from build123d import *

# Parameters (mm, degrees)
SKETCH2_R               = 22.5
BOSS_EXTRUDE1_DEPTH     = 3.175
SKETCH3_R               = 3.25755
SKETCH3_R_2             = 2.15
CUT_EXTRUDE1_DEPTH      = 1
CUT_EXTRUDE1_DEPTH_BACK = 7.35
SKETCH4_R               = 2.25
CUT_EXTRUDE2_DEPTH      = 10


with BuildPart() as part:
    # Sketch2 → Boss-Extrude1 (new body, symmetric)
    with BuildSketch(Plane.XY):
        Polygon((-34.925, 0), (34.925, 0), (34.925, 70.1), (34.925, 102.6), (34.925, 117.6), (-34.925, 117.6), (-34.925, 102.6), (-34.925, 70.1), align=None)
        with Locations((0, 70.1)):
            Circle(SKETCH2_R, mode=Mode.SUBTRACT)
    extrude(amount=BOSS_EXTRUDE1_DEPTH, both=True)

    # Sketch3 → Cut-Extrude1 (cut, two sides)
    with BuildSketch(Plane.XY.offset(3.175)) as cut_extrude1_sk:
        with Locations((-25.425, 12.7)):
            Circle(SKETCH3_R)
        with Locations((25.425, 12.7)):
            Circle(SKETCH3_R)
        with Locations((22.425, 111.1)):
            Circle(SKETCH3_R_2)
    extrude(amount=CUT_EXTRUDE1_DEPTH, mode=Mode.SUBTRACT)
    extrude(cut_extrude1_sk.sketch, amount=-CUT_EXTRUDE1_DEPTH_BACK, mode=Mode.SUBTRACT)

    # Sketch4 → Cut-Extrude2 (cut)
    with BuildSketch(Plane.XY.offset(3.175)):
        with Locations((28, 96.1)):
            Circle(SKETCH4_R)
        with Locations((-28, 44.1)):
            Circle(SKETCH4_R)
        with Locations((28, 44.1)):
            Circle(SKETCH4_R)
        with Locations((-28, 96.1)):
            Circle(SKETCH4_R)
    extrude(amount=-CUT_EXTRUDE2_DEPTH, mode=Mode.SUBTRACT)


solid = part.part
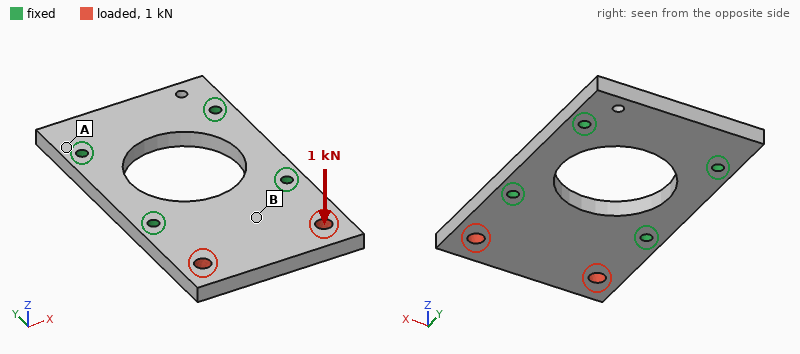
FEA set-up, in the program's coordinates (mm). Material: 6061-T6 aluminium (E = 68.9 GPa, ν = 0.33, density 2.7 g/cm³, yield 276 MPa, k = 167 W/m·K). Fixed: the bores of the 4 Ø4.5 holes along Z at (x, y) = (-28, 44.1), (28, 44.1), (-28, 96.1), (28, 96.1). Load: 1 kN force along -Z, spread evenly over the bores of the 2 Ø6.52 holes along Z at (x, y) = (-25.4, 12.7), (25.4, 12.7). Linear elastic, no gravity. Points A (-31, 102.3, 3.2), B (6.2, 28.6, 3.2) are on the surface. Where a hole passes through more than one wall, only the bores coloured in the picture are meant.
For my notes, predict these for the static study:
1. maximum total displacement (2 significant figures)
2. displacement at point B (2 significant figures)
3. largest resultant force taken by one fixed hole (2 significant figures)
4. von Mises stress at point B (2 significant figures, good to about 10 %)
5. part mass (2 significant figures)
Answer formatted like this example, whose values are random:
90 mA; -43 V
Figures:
0.23 mm; 0.063 mm; 550 N; 25 MPa; 110 g
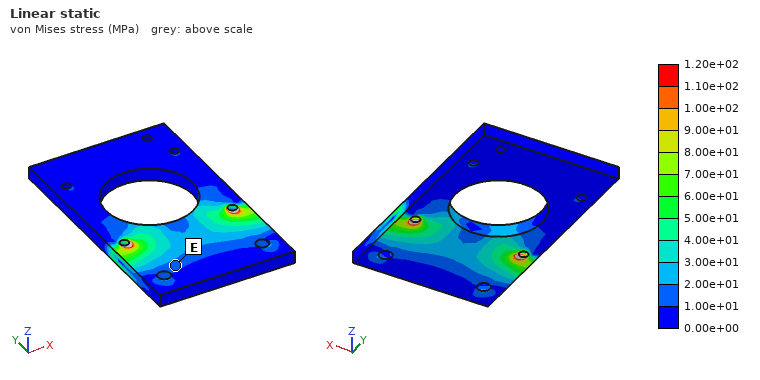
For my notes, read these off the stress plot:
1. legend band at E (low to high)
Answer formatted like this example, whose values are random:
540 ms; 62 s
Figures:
1.00e+01 to 2.00e+01 MPa
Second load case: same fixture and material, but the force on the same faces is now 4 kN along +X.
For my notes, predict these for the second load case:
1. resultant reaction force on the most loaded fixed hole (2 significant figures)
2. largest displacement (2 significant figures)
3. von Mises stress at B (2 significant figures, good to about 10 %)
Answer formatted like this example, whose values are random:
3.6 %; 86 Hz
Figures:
2.9 kN; 23 µm; 19 MPa
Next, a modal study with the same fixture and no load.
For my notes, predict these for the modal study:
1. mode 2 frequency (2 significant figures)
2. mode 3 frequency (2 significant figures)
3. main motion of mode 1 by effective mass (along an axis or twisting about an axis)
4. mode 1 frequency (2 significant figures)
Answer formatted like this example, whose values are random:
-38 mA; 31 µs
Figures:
4600 Hz; 6600 Hz; along Z; 2200 Hz
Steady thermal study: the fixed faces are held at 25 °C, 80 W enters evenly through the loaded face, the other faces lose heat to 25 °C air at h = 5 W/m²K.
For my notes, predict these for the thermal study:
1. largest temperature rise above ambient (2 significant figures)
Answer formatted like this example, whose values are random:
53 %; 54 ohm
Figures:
52 K
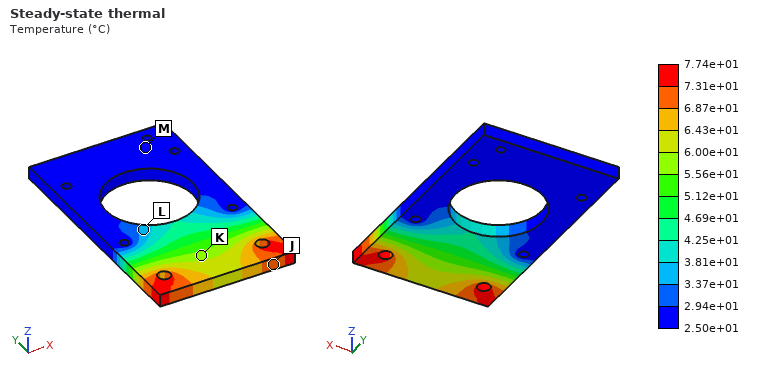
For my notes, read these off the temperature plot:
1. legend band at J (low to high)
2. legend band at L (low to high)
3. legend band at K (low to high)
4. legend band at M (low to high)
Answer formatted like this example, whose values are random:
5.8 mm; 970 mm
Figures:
6.87e+01 to 7.31e+01 °C; 3.37e+01 to 3.81e+01 °C; 5.56e+01 to 6.00e+01 °C; 2.50e+01 to 2.94e+01 °C
